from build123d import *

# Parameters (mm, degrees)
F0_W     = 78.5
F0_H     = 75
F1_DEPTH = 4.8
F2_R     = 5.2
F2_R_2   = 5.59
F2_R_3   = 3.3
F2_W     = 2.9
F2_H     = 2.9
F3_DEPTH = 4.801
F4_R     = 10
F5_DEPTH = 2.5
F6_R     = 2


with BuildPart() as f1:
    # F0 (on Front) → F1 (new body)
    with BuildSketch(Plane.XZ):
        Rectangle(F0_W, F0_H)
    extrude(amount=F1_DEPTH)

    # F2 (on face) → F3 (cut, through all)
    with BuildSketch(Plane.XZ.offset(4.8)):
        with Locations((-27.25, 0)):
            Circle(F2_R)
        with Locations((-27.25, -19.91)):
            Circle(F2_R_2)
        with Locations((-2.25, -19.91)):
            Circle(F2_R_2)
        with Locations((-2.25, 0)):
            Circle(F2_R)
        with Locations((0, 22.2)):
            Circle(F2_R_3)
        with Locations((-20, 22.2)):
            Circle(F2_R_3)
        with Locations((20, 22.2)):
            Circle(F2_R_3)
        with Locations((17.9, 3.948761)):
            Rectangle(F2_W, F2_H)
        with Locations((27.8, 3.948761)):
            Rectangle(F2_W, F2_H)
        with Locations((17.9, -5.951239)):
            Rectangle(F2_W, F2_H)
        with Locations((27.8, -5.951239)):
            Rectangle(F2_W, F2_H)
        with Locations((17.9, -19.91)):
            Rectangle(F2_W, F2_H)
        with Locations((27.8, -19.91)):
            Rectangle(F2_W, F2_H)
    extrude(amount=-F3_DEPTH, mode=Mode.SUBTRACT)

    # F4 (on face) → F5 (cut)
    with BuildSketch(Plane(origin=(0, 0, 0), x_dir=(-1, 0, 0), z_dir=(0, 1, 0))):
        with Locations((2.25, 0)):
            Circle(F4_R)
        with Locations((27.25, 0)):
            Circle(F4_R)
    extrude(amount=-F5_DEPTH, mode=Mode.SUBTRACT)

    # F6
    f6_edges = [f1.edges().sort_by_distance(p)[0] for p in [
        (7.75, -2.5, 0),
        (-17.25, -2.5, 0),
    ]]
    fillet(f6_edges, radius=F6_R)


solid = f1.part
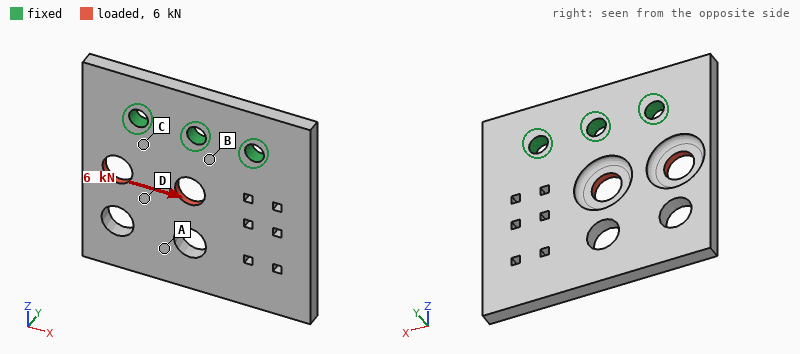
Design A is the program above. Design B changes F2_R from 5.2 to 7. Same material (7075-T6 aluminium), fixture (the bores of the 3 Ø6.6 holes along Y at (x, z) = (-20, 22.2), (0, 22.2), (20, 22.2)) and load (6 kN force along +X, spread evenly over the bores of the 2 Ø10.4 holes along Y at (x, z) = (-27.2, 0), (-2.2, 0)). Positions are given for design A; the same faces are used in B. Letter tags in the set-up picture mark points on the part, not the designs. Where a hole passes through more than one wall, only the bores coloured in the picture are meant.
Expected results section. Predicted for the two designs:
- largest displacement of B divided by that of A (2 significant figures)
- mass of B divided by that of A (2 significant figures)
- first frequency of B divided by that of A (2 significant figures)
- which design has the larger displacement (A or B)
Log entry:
1.2
0.99
0.98
B
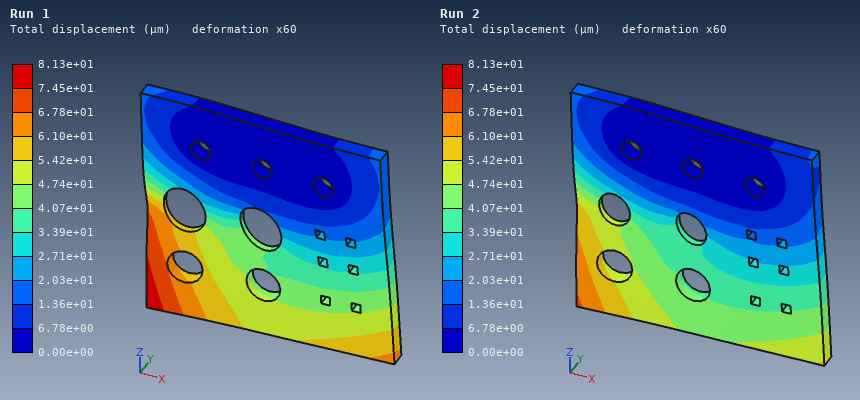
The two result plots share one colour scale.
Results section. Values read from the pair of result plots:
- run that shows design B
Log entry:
Run 1
